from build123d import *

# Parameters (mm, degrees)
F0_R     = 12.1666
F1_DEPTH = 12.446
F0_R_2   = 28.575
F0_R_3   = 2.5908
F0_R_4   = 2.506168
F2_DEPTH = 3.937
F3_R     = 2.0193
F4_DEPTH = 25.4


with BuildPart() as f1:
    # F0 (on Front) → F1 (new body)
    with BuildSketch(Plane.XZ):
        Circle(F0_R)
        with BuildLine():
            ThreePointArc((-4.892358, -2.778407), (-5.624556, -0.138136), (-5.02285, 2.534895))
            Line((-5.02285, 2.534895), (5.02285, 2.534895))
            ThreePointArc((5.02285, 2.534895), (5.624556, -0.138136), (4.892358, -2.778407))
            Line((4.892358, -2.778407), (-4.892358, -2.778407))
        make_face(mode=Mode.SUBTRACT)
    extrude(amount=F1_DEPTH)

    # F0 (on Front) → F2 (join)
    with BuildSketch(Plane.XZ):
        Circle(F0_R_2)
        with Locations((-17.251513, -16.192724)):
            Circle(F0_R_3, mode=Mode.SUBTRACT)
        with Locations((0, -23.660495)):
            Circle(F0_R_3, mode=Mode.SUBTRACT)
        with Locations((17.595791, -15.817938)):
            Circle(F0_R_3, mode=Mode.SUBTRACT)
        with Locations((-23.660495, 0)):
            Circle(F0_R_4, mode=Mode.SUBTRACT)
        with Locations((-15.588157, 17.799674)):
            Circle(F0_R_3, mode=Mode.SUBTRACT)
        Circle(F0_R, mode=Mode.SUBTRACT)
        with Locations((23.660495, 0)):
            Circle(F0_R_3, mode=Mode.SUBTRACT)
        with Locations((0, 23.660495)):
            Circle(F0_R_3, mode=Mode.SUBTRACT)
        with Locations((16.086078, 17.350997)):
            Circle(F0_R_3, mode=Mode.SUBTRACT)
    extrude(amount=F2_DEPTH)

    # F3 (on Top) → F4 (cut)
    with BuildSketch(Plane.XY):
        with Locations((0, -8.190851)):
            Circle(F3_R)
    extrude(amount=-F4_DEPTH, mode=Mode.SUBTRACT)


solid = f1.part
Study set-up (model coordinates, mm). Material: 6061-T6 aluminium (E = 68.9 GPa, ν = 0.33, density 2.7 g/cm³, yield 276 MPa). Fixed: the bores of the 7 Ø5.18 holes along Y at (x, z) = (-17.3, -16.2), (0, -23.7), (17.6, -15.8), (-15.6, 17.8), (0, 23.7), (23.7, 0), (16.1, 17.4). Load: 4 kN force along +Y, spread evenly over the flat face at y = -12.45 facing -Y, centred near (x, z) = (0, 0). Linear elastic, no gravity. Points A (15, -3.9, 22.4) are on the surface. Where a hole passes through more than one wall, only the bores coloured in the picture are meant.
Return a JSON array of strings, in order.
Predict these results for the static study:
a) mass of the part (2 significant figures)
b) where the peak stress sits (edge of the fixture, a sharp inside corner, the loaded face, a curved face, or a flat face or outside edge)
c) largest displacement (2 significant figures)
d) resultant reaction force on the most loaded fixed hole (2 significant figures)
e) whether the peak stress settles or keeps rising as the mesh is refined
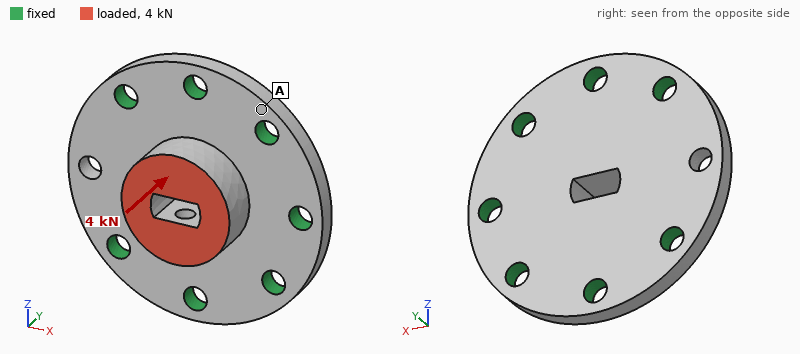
["34 g", "edge of the fixture", "30 µm", "840 N", "keeps rising"]
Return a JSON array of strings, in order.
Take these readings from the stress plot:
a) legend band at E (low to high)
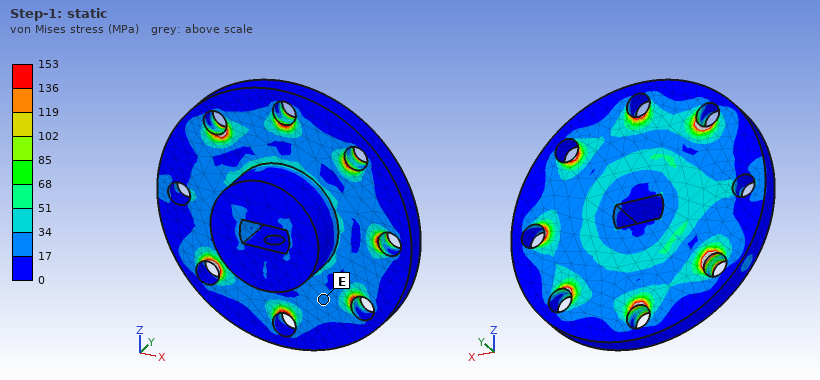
["17 to 34 MPa"]
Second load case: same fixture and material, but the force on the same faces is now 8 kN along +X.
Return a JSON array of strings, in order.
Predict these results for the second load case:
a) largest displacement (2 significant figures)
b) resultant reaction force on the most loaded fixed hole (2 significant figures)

["77 µm", "2.3 kN"]
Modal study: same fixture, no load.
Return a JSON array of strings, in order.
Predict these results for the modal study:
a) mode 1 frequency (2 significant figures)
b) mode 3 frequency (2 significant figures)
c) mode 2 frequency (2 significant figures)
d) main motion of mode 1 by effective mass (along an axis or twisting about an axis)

["15 kHz", "23 kHz", "17 kHz", "along Y"]
